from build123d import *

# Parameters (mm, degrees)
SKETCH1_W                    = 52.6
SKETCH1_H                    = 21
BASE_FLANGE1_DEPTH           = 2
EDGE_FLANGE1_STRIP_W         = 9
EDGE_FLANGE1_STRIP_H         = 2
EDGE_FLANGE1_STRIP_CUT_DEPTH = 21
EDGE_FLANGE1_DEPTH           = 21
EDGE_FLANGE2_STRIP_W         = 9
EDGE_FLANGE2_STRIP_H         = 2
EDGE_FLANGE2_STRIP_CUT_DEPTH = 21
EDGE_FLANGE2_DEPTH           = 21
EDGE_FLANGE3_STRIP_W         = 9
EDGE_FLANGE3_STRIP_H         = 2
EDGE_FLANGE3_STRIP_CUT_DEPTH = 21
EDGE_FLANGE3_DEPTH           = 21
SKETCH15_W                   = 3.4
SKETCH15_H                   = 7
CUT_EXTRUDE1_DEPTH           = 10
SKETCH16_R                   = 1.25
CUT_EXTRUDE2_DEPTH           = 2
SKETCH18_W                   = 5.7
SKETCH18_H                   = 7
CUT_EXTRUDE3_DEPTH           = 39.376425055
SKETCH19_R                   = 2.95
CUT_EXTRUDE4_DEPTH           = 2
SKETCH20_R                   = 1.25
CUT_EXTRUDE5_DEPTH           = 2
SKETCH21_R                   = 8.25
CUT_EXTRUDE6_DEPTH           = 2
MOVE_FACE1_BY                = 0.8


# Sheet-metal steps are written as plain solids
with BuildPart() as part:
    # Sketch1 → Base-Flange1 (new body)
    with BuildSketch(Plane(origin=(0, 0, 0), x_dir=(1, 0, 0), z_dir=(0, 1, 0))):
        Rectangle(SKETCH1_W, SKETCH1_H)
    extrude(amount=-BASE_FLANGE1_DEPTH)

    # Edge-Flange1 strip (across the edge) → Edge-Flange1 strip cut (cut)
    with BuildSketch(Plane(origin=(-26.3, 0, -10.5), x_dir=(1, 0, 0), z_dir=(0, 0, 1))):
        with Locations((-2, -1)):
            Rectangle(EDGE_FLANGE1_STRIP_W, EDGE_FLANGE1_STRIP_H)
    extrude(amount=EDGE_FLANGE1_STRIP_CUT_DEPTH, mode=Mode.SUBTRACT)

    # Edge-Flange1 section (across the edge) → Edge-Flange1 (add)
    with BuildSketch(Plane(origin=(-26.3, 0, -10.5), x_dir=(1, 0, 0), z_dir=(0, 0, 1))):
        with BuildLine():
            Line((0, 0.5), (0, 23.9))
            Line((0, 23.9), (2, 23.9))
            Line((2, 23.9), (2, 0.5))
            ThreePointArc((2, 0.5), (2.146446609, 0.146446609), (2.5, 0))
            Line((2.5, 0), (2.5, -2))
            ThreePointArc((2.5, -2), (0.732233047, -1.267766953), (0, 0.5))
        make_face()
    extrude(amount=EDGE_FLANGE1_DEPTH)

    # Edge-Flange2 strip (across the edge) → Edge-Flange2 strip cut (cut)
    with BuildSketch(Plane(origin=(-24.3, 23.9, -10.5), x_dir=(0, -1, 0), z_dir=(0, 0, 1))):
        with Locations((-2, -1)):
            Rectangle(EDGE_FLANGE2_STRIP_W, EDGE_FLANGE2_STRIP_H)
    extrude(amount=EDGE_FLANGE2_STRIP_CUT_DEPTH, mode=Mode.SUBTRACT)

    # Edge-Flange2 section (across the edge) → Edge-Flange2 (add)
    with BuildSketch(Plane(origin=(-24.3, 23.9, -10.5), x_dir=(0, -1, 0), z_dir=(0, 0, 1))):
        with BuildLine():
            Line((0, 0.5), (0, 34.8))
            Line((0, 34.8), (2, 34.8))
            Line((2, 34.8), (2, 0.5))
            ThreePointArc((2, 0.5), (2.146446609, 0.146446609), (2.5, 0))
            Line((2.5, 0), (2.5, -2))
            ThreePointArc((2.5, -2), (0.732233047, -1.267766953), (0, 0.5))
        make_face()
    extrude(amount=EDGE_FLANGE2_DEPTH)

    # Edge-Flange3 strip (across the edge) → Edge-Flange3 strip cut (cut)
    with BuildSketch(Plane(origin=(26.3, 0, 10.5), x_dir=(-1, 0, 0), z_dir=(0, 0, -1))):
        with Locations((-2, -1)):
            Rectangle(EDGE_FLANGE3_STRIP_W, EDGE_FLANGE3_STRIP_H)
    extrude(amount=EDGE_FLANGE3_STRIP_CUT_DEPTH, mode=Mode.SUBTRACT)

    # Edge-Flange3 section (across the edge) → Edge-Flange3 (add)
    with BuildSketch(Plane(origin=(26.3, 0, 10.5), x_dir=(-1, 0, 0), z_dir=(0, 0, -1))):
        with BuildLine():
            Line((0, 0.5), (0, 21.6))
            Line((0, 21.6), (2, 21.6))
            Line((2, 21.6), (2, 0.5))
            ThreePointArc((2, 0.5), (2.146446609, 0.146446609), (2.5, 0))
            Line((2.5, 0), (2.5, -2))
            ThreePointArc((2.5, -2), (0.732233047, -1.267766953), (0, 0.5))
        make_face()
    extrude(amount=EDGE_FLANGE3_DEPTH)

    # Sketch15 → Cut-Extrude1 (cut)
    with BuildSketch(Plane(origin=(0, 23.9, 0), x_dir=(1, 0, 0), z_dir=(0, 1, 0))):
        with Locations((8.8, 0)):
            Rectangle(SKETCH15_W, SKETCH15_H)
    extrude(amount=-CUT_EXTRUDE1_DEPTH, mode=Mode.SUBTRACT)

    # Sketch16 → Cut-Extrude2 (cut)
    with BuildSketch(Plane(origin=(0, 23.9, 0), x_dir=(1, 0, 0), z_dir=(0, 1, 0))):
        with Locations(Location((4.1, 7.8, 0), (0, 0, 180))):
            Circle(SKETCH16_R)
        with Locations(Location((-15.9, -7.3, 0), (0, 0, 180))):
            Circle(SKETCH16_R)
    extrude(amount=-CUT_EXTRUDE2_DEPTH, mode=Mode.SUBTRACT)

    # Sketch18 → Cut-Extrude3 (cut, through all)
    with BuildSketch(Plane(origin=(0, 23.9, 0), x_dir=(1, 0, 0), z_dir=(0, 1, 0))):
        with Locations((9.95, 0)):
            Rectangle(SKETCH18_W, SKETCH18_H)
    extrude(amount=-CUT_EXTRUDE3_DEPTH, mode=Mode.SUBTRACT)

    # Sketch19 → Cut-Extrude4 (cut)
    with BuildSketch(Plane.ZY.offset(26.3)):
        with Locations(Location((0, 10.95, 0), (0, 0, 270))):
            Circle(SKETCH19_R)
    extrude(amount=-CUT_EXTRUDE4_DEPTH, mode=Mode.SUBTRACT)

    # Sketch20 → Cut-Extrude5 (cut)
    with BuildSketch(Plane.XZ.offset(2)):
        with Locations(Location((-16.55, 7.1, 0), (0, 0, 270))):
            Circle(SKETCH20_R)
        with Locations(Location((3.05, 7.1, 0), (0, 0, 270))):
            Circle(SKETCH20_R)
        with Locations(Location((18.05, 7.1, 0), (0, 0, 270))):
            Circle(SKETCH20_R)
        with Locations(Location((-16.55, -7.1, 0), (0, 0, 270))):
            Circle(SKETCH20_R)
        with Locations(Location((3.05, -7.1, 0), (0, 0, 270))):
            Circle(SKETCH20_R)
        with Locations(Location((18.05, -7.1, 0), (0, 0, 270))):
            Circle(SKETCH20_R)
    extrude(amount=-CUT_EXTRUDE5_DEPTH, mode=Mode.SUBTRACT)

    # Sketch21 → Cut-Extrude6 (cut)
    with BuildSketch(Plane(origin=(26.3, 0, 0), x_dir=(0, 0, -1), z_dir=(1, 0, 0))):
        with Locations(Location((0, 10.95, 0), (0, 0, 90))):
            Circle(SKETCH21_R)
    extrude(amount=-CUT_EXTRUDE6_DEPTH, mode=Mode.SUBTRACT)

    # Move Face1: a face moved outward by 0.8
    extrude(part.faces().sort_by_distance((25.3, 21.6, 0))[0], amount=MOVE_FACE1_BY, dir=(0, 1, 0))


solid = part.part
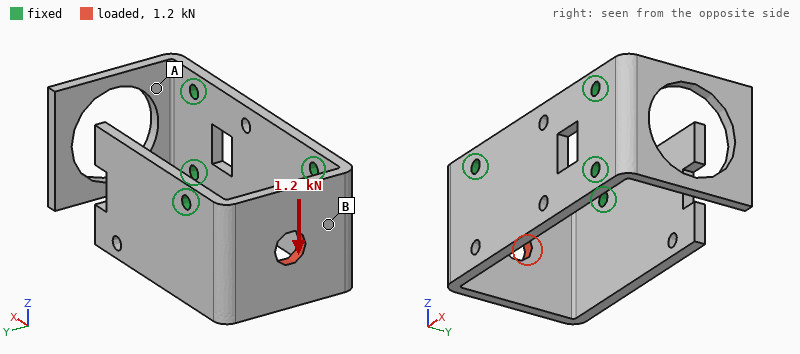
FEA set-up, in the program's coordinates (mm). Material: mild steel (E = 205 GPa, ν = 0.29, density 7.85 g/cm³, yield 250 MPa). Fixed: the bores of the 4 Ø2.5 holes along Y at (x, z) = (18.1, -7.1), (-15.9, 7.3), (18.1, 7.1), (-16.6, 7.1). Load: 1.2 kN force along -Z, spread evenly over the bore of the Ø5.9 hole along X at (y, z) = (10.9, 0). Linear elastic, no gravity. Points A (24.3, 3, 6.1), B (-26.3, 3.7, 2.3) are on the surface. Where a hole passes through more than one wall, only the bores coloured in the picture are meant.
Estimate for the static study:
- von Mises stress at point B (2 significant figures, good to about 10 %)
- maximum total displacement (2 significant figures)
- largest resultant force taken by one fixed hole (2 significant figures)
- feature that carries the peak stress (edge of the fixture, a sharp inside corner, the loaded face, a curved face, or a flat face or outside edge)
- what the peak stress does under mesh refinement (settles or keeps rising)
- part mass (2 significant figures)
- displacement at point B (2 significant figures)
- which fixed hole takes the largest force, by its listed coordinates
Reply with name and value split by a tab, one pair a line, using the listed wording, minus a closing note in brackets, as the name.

von Mises stress at point B	51 MPa
maximum total displacement	52 µm
largest resultant force taken by one fixed hole	750 N
feature that carries the peak stress	edge of the fixture
what the peak stress does under mesh refinement	keeps rising
part mass	38 g
displacement at point B	9.7 µm
which fixed hole takes the largest force, by its listed coordinates	(-16.6, 7.1)
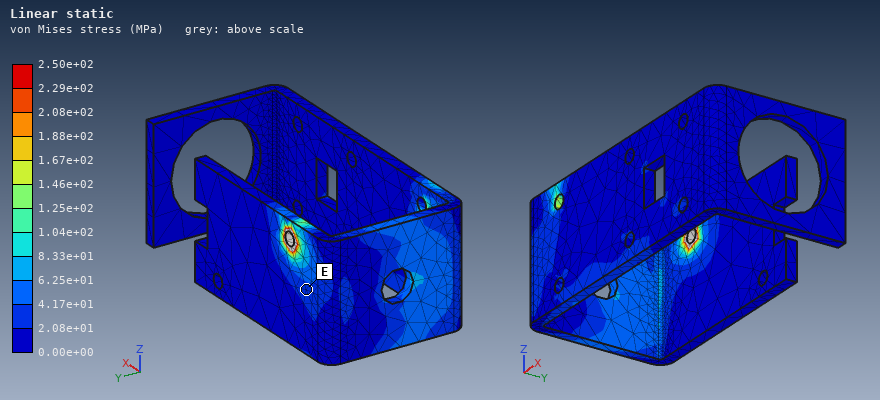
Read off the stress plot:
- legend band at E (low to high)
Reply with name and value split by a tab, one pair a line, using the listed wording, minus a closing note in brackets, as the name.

legend band at E	2.08e+01 to 4.17e+01 MPa
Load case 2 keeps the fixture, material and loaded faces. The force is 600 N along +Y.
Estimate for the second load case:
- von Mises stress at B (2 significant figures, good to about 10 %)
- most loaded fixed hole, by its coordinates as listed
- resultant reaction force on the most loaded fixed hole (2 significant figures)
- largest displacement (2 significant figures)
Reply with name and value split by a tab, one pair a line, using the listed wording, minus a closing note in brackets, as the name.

von Mises stress at B	42 MPa
most loaded fixed hole, by its coordinates as listed	(-16.6, 7.1)
resultant reaction force on the most loaded fixed hole	380 N
largest displacement	23 µm
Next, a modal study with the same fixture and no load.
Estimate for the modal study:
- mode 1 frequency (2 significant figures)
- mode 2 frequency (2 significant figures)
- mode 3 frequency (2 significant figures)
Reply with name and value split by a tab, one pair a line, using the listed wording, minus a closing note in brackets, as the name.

mode 1 frequency	2000 Hz
mode 2 frequency	2200 Hz
mode 3 frequency	4800 Hz
